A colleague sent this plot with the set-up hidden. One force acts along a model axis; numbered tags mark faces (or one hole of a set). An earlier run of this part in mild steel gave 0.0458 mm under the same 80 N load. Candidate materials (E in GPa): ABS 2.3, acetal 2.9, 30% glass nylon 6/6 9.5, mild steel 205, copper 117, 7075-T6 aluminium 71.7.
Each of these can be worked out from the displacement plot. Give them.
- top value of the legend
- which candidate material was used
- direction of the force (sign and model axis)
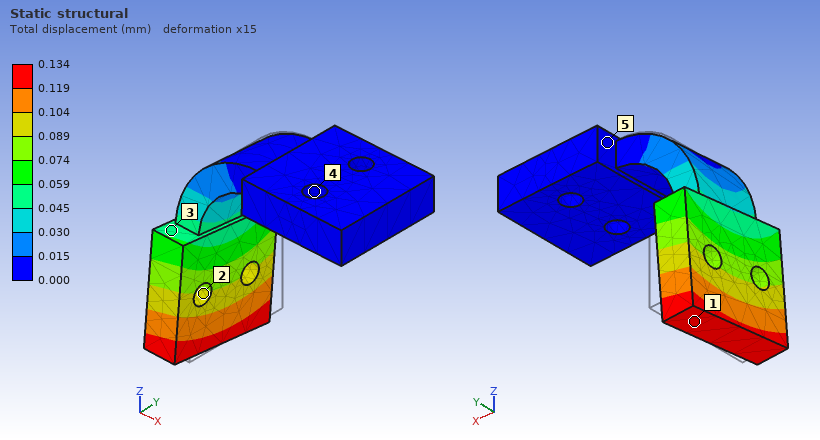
0.134 mm
7075-T6 aluminium
-Y
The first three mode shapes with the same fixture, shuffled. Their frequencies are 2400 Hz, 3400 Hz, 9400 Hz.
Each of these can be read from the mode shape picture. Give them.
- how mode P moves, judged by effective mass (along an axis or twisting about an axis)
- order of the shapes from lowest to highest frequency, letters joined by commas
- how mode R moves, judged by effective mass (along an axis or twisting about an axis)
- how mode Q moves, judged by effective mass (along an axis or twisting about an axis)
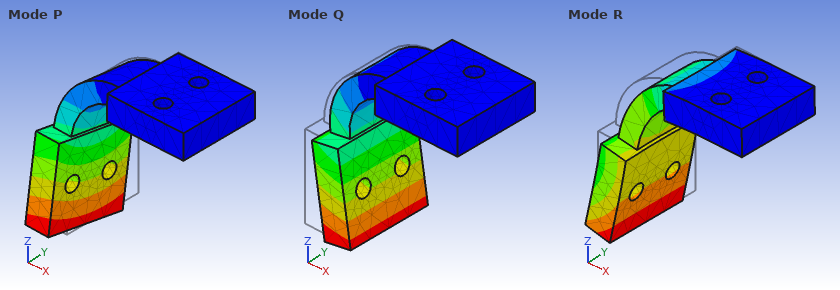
along Y
Q, P, R
along Z
along X
